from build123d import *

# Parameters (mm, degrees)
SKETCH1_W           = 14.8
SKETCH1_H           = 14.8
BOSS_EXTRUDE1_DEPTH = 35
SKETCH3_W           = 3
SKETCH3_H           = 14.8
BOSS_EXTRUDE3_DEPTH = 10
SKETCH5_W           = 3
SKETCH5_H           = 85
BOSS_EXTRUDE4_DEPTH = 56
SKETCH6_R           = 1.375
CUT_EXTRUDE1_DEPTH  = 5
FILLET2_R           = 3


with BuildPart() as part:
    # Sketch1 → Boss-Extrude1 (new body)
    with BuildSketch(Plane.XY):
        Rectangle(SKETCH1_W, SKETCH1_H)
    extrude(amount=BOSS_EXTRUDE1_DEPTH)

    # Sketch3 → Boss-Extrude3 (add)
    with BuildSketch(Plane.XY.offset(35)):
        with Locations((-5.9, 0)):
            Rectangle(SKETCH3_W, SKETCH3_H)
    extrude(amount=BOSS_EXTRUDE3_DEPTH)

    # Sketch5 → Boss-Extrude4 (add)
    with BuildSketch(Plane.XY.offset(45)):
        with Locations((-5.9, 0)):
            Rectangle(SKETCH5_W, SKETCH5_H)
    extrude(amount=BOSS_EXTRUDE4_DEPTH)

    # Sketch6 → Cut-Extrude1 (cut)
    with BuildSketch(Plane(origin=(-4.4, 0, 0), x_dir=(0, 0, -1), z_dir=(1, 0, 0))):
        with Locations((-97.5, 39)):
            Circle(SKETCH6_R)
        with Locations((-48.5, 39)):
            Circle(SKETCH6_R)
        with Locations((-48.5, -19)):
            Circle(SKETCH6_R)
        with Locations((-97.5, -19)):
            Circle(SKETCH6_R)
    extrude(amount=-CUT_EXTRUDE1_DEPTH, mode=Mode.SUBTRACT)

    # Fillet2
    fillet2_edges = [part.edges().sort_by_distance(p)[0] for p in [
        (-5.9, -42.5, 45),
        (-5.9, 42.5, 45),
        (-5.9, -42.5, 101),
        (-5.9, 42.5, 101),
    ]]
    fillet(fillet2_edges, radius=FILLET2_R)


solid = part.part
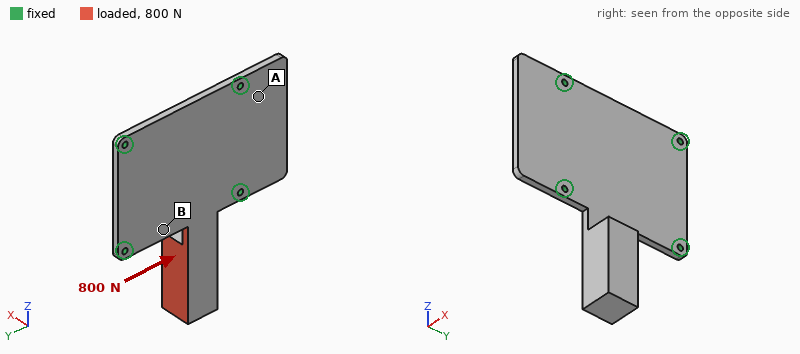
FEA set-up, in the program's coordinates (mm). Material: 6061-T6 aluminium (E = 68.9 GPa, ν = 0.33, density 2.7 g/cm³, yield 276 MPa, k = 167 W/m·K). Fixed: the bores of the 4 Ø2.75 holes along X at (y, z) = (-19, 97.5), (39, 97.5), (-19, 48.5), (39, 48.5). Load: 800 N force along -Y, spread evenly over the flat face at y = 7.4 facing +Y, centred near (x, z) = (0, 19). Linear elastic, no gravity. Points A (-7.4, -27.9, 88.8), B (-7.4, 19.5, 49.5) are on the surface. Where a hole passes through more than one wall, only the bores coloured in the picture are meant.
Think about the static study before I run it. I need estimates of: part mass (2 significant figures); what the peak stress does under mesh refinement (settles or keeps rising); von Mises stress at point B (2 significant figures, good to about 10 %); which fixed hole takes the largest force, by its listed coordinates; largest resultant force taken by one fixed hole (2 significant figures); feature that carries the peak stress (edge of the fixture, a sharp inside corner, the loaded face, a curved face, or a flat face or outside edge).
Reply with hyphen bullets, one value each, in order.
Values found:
- 60 g
- keeps rising
- 41 MPa
- (-19, 48.5)
- 740 N
- a sharp inside corner
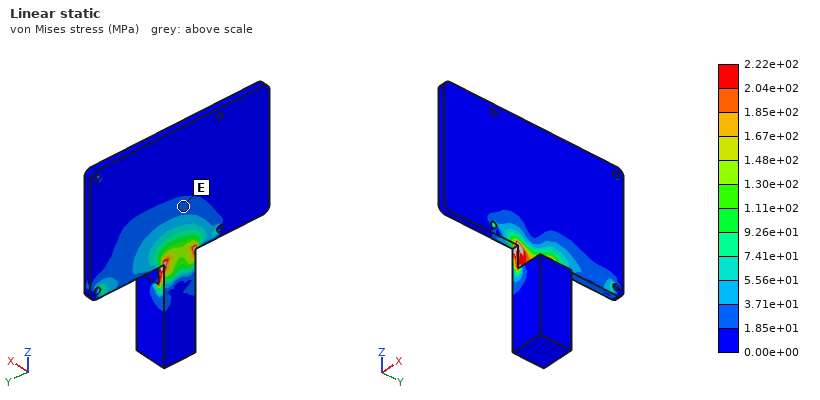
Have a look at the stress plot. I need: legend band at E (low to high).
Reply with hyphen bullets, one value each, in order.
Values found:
- 1.85e+01 to 3.71e+01 MPa
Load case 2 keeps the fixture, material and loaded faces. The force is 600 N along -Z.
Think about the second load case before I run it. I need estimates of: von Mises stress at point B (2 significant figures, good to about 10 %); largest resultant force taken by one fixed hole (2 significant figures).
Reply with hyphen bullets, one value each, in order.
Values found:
- 27 MPa
- 180 N
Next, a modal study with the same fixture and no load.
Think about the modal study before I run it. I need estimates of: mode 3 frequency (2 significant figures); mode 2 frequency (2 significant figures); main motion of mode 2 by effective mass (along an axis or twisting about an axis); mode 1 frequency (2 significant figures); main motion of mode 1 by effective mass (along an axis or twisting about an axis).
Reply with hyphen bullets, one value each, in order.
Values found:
- 2800 Hz
- 1600 Hz
- along Y
- 400 Hz
- along X
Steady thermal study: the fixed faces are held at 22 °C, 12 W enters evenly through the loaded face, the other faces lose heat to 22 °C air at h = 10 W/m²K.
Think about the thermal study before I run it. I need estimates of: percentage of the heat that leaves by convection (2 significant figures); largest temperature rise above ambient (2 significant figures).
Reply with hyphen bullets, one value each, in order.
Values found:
- 9.8 %
- 41 K
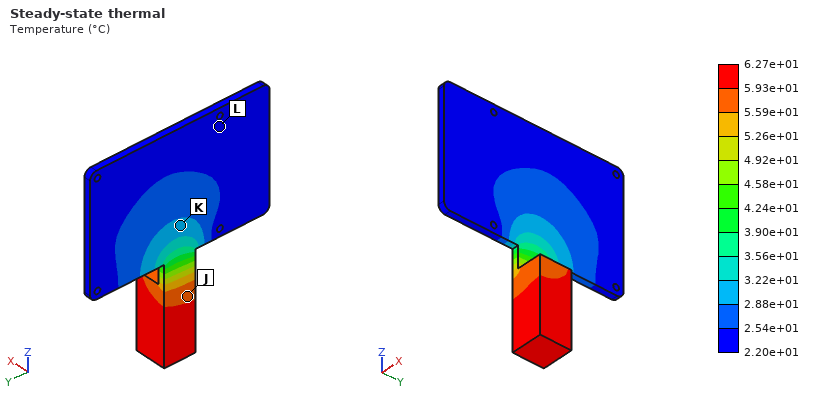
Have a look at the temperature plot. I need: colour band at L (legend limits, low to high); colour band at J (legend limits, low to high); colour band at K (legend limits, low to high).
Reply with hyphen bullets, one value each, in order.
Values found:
- 2.20e+01 to 2.54e+01 °C
- 5.59e+01 to 5.93e+01 °C
- 2.88e+01 to 3.22e+01 °C
